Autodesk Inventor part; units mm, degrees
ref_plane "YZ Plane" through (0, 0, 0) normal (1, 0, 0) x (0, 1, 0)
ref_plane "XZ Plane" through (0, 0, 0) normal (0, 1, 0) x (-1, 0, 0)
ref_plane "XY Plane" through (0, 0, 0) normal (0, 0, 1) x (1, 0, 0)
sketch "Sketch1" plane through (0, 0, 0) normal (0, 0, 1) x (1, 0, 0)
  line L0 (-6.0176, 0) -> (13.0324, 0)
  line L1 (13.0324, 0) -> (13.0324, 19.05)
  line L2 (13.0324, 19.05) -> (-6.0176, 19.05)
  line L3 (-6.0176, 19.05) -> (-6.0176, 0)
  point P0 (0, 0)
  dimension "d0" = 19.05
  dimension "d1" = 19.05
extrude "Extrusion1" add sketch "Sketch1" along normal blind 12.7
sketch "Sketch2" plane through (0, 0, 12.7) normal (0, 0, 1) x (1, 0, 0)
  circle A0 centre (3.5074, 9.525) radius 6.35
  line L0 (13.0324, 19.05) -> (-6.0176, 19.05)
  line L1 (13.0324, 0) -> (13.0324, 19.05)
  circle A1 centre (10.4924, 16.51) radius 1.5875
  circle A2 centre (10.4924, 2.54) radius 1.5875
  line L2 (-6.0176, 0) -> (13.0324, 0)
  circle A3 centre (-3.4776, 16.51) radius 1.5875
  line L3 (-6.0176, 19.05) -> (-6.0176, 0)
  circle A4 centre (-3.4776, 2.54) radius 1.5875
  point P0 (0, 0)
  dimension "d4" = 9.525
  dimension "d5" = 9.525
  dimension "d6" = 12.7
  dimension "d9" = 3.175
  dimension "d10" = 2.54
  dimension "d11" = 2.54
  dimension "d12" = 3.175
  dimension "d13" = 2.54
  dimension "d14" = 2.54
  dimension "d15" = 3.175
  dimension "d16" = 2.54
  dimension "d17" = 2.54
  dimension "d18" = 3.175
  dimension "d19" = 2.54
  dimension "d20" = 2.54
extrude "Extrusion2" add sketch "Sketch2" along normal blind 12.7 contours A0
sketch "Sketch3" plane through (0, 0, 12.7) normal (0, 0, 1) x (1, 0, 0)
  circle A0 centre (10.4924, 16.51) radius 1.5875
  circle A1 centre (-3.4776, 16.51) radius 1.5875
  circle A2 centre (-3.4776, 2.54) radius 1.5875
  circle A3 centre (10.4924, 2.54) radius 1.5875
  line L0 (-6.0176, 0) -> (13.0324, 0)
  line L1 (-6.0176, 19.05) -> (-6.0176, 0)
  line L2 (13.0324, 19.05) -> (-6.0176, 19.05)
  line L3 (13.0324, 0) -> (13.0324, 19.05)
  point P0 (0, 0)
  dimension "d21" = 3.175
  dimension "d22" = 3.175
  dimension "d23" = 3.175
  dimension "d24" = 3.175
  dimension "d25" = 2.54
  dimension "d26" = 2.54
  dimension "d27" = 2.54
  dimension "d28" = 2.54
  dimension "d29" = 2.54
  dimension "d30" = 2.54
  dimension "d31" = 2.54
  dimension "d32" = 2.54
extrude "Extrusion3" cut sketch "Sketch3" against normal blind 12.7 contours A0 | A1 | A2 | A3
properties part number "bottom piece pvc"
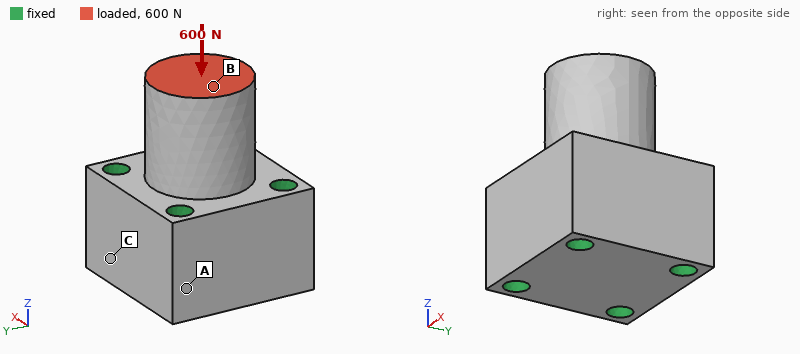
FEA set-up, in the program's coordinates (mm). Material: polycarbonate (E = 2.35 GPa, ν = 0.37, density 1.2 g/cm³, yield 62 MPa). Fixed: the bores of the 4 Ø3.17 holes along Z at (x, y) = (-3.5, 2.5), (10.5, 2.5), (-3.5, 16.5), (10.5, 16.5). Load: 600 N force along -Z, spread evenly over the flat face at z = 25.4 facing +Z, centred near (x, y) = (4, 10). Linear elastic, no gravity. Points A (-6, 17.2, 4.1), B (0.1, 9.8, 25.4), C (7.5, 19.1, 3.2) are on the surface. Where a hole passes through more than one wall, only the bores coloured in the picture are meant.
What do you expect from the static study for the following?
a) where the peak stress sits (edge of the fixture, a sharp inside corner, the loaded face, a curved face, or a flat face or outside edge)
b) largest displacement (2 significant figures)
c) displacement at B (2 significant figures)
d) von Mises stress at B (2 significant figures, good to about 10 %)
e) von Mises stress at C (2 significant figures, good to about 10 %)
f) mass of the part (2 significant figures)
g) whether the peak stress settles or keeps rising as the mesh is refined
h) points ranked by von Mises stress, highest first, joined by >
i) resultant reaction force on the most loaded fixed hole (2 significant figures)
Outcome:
edge of the fixture
37 µm
37 µm
4.8 MPa
1.5 MPa
7.0 g
keeps rising
B > C > A
160 N
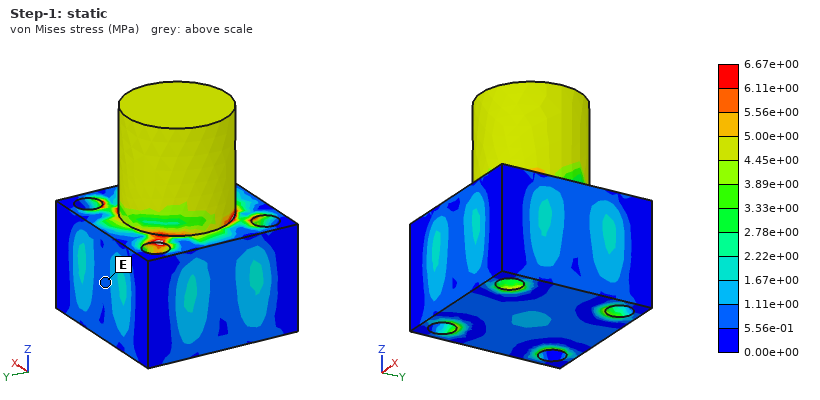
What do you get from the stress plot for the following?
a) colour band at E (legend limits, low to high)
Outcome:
5.56e-01 to 1.11e+00 MPa
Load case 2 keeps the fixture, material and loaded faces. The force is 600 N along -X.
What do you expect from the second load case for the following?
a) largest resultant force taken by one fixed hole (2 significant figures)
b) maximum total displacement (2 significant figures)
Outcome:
400 N
0.37 mm
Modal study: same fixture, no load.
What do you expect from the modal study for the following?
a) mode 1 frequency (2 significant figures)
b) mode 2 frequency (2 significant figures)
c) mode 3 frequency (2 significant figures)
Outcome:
8100 Hz
8100 Hz
15 kHz
